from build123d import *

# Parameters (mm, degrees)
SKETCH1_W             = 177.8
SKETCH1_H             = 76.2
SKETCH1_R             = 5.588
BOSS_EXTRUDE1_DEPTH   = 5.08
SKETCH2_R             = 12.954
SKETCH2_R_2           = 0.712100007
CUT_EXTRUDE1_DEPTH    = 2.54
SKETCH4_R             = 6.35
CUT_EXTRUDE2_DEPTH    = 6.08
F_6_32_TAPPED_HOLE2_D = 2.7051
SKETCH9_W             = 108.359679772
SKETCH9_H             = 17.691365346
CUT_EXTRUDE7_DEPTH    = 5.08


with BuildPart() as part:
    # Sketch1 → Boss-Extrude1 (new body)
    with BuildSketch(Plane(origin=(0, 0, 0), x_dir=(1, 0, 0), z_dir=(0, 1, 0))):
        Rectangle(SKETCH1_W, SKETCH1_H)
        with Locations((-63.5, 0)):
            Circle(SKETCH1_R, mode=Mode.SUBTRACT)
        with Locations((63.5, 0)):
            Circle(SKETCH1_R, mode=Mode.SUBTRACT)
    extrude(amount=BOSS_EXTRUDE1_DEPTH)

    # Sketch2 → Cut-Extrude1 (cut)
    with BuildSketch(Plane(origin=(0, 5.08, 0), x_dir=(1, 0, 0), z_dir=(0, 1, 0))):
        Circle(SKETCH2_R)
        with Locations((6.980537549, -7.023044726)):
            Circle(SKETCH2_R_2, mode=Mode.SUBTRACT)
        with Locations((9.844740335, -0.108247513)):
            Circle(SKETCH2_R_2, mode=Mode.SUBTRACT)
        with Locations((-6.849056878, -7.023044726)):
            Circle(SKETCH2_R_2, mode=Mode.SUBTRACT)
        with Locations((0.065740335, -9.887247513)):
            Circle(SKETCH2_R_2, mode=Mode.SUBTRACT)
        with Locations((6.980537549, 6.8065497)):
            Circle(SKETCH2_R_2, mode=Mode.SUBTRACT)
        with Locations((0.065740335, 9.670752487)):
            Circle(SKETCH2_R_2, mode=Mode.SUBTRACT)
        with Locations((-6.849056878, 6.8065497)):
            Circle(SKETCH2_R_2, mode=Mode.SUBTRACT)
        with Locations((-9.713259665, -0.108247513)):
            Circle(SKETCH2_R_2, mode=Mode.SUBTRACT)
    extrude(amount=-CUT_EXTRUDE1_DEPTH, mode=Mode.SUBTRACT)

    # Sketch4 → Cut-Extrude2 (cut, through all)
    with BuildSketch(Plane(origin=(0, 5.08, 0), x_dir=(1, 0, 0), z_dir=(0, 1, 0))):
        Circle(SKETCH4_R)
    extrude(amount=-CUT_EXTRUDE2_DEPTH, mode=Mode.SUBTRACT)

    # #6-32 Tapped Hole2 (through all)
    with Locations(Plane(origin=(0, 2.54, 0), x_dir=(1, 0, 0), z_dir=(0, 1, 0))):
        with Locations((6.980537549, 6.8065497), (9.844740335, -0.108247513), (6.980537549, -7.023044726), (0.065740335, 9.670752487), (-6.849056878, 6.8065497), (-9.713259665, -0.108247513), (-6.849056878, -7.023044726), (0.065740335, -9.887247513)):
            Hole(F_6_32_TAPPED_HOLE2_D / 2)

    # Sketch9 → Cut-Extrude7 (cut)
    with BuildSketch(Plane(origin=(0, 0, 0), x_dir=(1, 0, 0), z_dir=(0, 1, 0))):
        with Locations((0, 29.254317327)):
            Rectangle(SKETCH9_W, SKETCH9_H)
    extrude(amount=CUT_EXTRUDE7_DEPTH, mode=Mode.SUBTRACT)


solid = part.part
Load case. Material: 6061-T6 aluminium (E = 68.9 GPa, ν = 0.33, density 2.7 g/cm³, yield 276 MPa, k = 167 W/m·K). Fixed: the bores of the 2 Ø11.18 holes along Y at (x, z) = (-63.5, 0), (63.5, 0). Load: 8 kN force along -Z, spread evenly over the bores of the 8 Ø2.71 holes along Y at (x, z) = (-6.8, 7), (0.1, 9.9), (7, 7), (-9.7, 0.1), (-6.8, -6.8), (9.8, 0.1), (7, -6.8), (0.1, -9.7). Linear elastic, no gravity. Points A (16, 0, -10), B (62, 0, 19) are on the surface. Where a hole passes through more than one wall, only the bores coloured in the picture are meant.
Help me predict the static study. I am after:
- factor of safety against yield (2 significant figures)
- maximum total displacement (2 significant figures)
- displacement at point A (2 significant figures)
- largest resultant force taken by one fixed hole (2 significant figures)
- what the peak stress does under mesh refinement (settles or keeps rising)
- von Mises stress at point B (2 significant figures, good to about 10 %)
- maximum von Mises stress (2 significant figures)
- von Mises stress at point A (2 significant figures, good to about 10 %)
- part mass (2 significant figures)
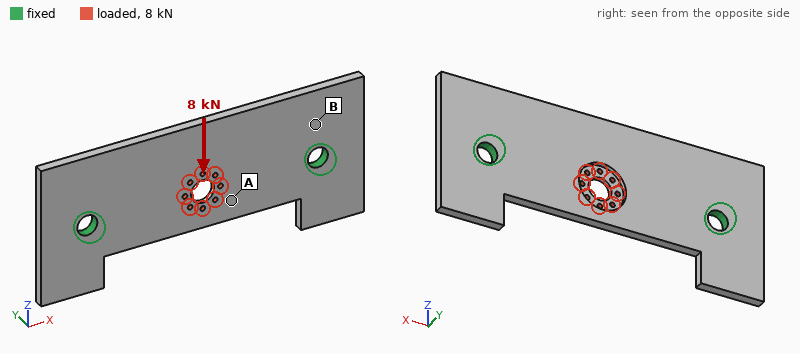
1.7
0.14 mm
0.090 mm
4.5 kN
settles
19 MPa
160 MPa
45 MPa
150 g
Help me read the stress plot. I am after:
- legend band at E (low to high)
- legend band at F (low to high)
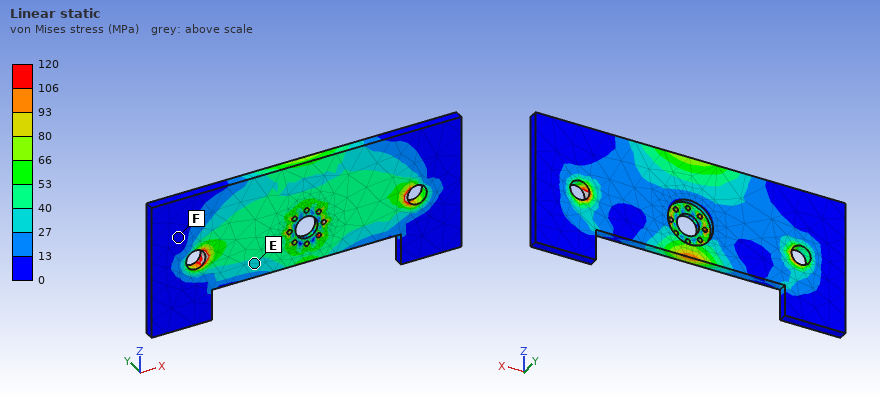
27 to 40 MPa
0 to 13 MPa
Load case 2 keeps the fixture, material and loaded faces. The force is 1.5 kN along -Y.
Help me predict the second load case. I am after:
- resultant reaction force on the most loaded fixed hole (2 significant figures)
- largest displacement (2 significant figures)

930 N
0.49 mm
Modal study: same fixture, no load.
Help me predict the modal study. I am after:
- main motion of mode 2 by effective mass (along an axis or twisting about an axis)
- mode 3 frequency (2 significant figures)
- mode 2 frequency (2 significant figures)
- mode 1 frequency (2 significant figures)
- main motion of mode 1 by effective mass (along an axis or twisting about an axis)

twisting about X
3100 Hz
2300 Hz
1500 Hz
along Y
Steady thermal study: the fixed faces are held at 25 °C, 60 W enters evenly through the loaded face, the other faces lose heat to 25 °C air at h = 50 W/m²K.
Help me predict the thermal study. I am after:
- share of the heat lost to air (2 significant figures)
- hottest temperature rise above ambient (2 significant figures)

26 %
46 K
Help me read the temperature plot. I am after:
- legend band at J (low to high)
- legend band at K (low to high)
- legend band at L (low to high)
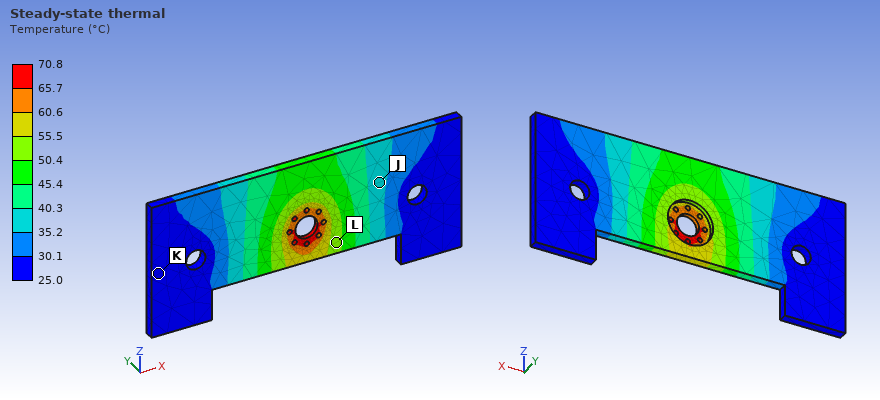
35.2 to 40.3 °C
25.0 to 30.1 °C
50.4 to 55.5 °C
